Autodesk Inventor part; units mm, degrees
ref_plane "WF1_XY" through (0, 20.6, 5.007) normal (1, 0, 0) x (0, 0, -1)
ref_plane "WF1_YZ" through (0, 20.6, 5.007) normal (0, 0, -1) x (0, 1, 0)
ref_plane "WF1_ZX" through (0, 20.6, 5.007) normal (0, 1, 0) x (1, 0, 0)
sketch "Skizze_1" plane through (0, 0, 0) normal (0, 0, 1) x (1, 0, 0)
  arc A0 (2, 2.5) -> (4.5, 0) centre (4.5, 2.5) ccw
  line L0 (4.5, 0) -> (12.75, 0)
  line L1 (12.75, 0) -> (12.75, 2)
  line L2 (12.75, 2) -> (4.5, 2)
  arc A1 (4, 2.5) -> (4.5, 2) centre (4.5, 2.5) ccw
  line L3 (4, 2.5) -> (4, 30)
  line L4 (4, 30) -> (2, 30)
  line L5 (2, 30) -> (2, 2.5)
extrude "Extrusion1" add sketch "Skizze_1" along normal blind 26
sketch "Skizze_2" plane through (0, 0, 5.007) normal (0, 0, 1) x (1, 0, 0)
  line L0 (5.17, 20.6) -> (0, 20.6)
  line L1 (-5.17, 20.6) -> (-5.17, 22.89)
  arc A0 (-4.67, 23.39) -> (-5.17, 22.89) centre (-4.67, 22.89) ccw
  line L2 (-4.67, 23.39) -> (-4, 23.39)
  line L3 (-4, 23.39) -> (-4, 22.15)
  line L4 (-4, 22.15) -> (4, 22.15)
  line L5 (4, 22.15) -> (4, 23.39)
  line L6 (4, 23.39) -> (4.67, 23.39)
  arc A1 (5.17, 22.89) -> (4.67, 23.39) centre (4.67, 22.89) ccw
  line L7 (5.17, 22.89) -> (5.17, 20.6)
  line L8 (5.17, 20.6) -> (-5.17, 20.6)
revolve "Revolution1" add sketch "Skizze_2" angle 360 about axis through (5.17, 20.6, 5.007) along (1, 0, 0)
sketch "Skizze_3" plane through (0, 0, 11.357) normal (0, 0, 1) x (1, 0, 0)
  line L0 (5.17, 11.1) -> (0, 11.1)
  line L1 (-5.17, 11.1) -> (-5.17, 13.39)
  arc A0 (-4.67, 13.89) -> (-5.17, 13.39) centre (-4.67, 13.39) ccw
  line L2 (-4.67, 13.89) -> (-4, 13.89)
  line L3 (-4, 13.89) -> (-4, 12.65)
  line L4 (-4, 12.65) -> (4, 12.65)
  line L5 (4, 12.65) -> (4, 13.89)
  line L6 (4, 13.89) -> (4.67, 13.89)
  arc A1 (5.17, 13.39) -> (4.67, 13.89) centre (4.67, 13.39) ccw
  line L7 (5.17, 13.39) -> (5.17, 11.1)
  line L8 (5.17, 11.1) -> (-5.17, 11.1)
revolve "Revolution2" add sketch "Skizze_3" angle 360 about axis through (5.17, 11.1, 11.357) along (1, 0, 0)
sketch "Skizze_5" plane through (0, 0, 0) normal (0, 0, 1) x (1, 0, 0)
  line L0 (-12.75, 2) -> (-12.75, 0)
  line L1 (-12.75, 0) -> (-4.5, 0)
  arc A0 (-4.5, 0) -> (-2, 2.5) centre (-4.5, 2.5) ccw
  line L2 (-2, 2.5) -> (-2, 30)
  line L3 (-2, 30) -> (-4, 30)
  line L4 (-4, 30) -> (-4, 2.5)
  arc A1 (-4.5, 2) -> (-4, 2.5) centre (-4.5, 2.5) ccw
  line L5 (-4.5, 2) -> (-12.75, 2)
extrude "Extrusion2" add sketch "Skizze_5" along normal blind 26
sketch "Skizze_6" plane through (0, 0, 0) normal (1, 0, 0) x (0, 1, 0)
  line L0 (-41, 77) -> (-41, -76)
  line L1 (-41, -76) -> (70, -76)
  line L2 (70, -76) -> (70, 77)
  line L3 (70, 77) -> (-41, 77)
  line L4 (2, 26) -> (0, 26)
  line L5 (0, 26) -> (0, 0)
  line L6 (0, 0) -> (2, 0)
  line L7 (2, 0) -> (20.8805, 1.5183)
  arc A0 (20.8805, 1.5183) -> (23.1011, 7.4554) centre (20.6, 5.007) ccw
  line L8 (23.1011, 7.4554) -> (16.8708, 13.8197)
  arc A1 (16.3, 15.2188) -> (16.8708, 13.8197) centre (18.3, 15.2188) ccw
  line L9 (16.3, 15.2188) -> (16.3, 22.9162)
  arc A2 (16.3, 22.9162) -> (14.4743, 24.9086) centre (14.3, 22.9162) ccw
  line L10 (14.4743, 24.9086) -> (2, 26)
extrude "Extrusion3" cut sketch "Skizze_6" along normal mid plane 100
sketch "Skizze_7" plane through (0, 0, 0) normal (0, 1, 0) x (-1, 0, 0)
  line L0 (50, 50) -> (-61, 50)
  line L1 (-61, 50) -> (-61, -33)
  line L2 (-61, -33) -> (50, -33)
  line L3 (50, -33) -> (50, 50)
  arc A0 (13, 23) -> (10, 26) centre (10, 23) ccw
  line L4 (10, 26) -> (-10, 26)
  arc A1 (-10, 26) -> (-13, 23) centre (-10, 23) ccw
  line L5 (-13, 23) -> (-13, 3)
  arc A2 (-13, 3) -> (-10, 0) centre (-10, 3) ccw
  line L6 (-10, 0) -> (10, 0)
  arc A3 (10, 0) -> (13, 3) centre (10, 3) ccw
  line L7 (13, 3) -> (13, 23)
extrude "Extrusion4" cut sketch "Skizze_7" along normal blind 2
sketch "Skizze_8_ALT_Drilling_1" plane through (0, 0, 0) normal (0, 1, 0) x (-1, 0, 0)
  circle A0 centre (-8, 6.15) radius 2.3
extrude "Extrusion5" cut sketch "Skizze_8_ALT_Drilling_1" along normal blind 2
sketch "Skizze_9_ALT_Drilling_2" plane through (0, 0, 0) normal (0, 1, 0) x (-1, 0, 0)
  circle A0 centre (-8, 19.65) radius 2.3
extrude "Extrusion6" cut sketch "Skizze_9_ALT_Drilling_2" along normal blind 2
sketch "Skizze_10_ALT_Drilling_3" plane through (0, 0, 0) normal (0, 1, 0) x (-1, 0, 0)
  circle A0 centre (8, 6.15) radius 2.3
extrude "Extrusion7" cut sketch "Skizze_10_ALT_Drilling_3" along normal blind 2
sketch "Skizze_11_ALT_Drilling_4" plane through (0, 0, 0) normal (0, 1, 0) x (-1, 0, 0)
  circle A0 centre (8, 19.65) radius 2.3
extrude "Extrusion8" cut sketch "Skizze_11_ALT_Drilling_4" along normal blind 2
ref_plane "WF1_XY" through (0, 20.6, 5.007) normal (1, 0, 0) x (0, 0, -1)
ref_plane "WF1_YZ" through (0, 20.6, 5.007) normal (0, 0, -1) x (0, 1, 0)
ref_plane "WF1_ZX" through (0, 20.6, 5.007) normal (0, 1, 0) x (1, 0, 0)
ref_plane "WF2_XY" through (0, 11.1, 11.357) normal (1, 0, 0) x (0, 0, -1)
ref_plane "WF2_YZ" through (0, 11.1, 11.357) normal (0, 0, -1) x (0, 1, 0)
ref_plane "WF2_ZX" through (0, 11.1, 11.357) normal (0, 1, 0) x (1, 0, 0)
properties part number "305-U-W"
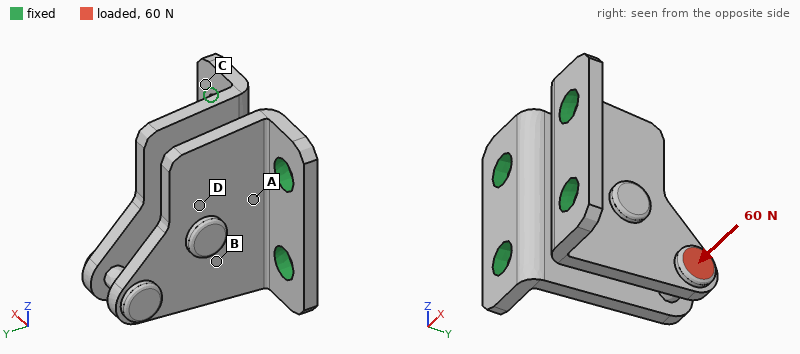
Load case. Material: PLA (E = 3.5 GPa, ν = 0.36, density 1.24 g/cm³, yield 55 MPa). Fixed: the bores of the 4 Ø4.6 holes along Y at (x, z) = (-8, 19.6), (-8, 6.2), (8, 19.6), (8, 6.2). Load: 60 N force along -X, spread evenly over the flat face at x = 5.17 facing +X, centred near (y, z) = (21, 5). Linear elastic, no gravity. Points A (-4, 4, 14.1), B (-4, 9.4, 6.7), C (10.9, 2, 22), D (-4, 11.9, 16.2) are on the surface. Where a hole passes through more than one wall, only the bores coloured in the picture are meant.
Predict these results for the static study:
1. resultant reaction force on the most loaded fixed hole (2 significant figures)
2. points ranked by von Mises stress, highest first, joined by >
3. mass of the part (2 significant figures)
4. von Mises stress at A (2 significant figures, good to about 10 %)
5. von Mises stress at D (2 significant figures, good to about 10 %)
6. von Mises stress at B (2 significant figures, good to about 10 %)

60 N
A > B > D > C
3.4 g
12 MPa
4.7 MPa
8.4 MPa
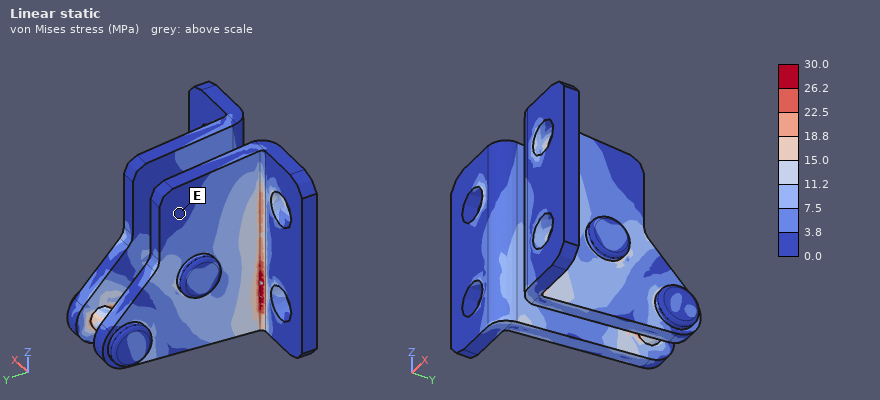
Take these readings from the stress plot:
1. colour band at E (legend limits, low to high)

0.0 to 3.8 MPa
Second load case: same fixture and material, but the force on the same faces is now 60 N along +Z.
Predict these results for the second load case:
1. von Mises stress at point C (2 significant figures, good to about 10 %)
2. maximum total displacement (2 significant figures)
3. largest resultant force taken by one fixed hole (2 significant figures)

2.2 MPa
0.26 mm
72 N
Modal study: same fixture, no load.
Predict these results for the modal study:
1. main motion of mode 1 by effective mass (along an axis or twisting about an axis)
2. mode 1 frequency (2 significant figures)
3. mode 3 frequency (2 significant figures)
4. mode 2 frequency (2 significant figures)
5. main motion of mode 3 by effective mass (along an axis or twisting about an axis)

along X
2400 Hz
4000 Hz
3300 Hz
along Z
